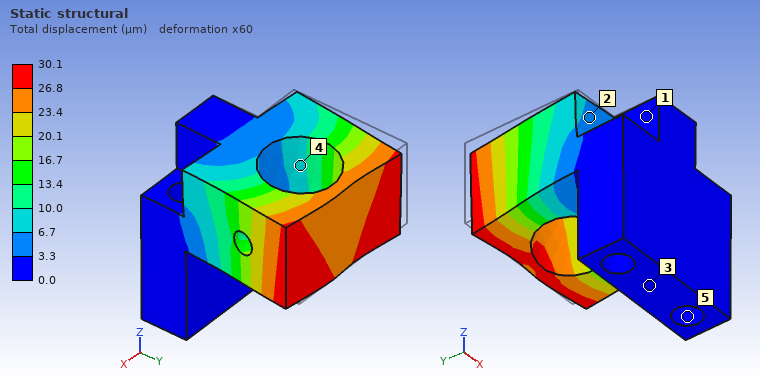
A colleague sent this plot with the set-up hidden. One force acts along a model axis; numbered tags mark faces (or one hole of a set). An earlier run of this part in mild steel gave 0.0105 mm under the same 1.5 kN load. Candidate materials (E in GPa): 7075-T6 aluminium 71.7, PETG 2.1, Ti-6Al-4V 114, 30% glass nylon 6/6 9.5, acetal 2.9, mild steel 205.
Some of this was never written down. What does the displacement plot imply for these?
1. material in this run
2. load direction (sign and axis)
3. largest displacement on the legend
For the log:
7075-T6 aluminium
+X
30.1 µm
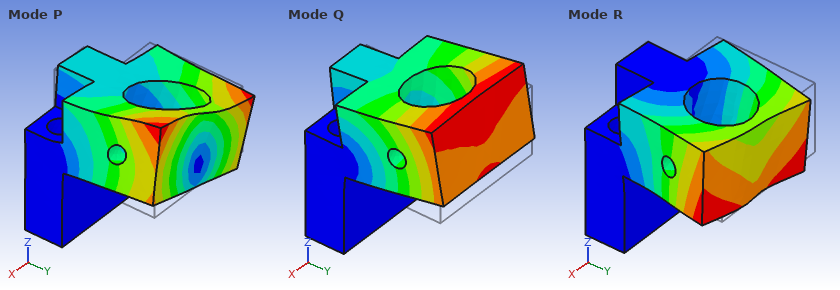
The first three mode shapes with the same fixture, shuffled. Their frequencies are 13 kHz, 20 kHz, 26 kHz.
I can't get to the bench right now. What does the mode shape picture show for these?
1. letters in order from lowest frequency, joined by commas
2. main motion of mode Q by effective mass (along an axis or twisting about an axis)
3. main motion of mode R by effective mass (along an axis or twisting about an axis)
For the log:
Q, R, P
along Z
along X
